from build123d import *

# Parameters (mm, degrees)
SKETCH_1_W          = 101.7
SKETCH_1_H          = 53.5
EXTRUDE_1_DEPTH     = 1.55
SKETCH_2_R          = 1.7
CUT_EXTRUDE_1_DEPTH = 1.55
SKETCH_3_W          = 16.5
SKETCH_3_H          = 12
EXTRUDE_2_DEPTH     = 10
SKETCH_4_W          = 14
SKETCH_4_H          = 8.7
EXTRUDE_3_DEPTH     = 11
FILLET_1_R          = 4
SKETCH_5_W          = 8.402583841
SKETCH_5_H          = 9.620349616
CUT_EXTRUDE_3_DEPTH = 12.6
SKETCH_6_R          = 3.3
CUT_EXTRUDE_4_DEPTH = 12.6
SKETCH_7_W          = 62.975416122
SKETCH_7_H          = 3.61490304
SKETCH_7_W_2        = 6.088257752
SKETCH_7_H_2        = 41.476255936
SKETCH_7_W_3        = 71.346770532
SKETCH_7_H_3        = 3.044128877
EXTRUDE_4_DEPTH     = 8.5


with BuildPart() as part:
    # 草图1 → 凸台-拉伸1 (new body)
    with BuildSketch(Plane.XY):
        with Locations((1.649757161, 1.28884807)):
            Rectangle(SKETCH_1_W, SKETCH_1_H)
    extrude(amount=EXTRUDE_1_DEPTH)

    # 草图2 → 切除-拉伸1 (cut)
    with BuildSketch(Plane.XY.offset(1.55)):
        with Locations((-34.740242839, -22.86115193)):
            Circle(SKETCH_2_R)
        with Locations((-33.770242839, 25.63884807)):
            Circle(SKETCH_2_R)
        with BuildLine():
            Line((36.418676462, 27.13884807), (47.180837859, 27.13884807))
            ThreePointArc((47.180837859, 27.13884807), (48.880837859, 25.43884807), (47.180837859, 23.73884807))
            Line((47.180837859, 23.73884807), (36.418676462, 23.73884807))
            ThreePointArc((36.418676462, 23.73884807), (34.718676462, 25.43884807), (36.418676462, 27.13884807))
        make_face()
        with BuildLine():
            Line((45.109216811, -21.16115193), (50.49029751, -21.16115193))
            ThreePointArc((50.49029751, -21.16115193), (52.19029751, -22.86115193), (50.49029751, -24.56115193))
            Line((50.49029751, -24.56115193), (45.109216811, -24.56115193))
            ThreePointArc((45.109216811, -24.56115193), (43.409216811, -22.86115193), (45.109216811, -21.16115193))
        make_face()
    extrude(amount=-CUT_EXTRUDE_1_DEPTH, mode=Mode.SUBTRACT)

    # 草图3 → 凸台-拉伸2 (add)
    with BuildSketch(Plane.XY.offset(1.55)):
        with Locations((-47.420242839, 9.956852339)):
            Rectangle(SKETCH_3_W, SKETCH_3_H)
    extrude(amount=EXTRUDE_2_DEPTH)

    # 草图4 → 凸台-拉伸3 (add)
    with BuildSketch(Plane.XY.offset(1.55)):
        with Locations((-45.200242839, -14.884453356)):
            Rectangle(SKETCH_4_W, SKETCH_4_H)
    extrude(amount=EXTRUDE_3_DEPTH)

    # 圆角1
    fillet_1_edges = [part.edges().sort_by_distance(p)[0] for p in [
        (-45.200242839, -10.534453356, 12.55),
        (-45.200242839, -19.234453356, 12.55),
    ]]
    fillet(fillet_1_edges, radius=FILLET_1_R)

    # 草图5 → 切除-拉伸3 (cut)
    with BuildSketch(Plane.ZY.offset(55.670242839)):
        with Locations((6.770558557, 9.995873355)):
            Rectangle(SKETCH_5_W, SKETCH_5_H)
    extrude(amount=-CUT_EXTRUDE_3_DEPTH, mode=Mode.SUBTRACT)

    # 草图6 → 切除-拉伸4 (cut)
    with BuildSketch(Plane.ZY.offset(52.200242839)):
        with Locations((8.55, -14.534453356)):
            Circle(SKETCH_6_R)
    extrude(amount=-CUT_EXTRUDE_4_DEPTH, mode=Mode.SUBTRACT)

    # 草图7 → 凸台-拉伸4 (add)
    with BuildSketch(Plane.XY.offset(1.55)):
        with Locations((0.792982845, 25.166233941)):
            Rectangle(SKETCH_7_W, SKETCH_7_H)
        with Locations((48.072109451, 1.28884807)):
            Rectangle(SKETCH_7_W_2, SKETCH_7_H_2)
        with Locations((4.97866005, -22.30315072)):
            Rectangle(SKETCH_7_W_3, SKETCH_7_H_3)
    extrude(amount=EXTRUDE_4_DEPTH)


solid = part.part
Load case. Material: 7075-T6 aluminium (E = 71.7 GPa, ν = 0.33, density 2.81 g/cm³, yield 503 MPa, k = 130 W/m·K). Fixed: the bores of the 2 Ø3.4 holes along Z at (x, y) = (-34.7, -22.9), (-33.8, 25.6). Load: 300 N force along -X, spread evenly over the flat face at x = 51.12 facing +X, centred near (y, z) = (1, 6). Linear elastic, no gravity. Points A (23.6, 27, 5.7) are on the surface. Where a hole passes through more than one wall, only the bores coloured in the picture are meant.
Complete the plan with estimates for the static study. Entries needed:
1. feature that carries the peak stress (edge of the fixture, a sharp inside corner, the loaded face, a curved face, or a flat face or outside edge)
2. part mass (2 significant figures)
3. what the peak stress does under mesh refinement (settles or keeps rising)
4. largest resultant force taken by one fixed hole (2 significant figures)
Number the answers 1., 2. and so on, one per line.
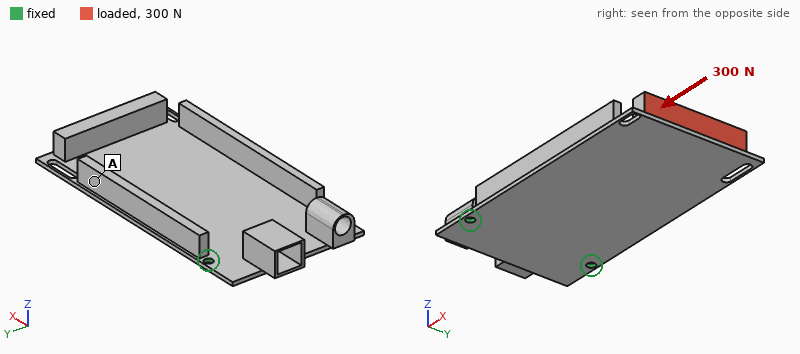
1. edge of the fixture
2. 45 g
3. keeps rising
4. 150 N
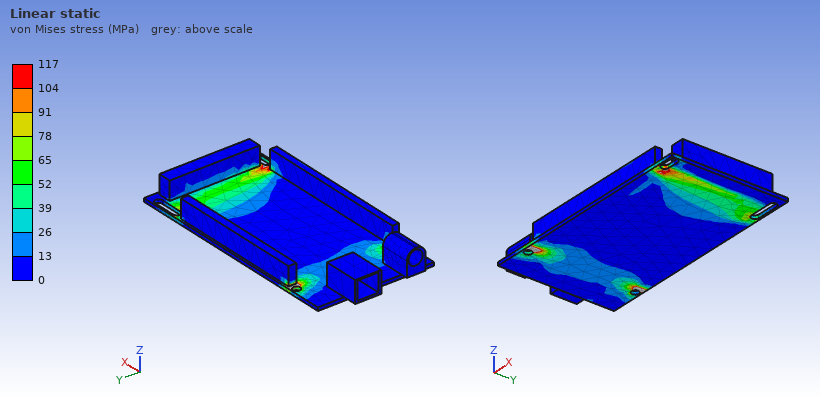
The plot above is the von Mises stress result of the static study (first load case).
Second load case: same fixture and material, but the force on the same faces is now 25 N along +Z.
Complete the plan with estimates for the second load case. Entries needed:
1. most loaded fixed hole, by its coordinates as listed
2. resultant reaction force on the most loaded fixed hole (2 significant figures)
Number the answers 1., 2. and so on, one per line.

1. (-33.8, 25.6)
2. 15 N
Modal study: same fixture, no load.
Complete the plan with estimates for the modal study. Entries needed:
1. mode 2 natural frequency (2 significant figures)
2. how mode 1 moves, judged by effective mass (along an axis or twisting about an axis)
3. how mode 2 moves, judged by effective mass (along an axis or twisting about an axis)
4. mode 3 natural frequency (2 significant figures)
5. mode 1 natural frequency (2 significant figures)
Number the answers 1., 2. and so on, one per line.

1. 630 Hz
2. along Z
3. twisting about X
4. 1700 Hz
5. 180 Hz
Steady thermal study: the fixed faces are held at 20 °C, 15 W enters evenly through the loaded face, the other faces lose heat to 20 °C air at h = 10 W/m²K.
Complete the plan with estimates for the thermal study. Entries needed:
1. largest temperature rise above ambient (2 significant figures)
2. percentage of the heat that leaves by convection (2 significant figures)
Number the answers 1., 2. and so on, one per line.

1. 75 K
2. 32 %
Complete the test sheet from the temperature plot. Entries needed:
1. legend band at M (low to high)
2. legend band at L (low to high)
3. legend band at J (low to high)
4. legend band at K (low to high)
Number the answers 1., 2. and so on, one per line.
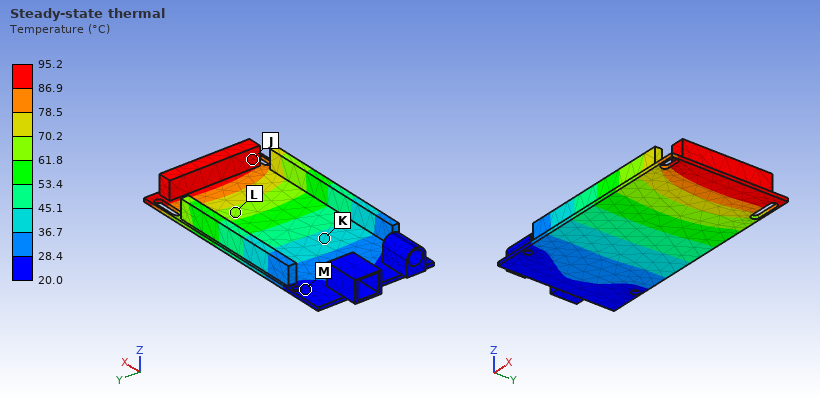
1. 20.0 to 28.4 °C
2. 61.8 to 70.2 °C
3. 86.9 to 95.2 °C
4. 36.7 to 45.1 °C
